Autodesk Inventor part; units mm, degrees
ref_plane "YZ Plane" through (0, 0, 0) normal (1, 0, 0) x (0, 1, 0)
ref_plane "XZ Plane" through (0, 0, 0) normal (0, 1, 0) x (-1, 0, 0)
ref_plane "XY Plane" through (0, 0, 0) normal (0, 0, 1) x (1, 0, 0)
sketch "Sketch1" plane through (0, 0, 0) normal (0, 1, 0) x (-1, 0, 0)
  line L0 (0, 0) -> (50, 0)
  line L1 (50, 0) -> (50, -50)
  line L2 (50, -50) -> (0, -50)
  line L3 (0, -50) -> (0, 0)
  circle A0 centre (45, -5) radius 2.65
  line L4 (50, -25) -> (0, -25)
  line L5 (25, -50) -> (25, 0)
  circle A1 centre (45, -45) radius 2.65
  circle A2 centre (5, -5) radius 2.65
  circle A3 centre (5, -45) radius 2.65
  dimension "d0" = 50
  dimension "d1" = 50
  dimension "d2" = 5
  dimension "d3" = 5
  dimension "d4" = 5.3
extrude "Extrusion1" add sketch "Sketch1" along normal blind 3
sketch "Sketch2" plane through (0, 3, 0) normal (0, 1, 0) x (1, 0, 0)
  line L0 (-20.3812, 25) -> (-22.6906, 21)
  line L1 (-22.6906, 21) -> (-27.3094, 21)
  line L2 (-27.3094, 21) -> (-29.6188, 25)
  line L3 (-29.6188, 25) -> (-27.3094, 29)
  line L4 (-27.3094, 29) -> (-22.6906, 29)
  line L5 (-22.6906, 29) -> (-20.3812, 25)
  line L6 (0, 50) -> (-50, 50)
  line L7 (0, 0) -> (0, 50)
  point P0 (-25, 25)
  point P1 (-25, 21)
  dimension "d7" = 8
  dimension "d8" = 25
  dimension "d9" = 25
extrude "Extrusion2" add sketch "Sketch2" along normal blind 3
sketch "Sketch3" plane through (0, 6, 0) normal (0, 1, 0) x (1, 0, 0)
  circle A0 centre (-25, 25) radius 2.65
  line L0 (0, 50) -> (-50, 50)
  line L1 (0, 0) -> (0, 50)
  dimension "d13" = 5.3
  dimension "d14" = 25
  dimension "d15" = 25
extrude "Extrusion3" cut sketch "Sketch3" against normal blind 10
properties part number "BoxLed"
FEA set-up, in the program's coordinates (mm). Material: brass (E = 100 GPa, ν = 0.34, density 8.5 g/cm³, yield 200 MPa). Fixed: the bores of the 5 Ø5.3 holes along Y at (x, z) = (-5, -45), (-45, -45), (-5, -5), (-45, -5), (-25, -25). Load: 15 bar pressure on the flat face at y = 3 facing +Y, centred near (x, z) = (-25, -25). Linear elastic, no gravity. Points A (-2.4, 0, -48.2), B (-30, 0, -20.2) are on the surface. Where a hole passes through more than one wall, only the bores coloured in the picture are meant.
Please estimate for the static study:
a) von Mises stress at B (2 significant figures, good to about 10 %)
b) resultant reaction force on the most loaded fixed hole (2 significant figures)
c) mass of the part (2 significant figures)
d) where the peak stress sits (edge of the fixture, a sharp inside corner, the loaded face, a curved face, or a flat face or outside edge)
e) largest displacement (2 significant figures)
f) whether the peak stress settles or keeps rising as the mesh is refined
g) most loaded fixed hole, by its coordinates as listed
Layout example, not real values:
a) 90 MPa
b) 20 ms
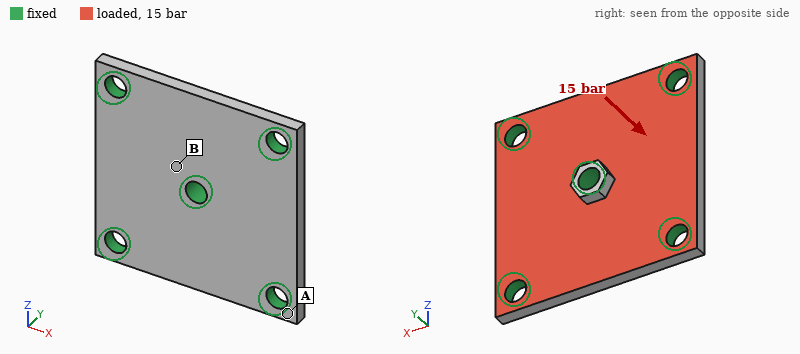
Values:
a) 33 MPa
b) 1.2 kN
c) 62 g
d) edge of the fixture
e) 26 µm
f) keeps rising
g) (-25, -25)
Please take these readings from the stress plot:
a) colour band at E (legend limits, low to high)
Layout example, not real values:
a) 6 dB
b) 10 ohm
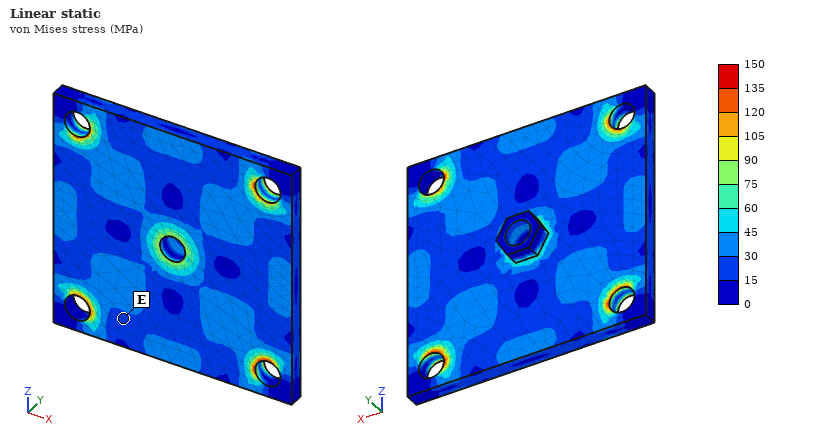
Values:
a) 15 to 30 MPa
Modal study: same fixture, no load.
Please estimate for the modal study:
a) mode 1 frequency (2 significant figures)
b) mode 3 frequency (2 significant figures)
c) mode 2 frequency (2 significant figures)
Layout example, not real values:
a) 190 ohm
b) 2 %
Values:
a) 8800 Hz
b) 9300 Hz
c) 9300 Hz
